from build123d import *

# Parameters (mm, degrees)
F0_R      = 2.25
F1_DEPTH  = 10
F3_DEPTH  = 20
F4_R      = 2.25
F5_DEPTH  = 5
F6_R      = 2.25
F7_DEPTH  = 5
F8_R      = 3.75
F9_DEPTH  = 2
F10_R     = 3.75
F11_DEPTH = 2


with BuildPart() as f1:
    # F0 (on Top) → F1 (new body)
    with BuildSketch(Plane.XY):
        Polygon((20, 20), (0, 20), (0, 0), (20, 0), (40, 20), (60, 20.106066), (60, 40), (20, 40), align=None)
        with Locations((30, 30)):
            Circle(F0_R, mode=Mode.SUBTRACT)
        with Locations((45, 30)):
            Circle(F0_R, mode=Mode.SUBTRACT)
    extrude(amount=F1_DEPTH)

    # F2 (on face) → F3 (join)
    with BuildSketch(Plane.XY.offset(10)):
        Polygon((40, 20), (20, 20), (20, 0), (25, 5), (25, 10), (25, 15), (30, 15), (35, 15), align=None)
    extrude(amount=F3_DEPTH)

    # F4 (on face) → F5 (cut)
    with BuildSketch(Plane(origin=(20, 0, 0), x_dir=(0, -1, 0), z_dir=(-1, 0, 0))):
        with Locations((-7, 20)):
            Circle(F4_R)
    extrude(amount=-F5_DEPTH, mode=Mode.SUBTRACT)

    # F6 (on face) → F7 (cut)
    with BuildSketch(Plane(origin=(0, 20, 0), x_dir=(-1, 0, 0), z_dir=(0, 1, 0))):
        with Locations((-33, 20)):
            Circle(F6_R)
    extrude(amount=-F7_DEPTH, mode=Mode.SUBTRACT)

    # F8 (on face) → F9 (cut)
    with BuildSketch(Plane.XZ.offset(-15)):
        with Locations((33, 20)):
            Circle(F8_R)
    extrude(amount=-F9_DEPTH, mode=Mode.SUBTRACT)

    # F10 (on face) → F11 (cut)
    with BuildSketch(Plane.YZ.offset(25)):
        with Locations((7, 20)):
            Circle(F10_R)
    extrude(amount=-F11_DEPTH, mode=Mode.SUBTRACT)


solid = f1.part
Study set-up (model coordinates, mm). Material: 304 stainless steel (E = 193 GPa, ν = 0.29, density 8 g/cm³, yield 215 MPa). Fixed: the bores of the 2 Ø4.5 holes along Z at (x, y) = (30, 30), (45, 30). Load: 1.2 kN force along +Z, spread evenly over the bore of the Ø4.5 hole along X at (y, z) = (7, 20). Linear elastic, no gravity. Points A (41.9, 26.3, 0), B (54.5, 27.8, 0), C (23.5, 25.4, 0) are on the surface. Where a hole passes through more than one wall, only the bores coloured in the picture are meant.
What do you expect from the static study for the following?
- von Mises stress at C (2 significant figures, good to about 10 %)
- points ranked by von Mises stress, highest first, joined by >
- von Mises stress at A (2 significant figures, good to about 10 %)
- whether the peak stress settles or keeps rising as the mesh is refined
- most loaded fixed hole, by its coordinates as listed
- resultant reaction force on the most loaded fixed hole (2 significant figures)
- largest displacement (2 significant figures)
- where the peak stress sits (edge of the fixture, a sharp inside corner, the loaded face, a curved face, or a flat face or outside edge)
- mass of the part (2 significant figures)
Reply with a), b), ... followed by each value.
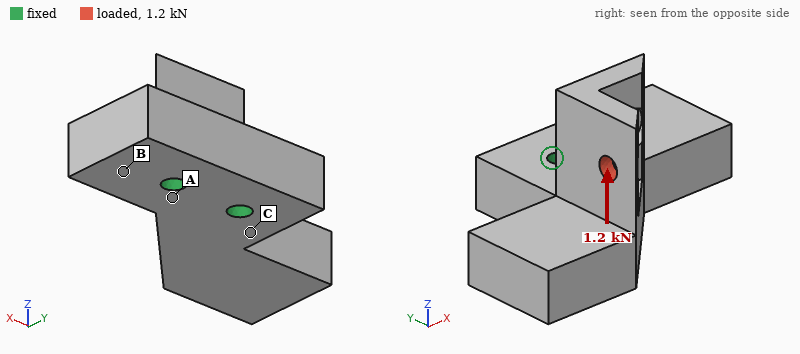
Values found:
a) 60 MPa
b) C > A > B
c) 40 MPa
d) keeps rising
e) (30, 30)
f) 1.4 kN
g) 43 µm
h) edge of the fixture
i) 130 g
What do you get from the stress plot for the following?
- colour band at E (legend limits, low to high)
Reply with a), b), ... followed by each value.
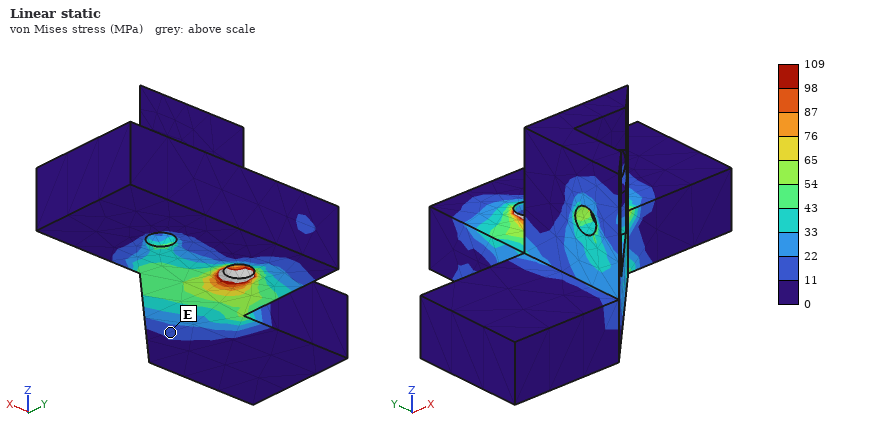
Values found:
a) 11 to 22 MPa
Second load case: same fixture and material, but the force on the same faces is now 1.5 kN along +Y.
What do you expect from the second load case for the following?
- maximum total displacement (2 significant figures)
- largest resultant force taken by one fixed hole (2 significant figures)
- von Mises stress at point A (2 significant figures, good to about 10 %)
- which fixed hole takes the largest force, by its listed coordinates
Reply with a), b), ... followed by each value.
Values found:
a) 52 µm
b) 2.1 kN
c) 45 MPa
d) (30, 30)
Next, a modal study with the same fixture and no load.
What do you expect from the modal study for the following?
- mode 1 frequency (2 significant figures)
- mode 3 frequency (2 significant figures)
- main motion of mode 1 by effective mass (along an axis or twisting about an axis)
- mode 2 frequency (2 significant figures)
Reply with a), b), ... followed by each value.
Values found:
a) 4300 Hz
b) 7900 Hz
c) along Z
d) 6700 Hz
